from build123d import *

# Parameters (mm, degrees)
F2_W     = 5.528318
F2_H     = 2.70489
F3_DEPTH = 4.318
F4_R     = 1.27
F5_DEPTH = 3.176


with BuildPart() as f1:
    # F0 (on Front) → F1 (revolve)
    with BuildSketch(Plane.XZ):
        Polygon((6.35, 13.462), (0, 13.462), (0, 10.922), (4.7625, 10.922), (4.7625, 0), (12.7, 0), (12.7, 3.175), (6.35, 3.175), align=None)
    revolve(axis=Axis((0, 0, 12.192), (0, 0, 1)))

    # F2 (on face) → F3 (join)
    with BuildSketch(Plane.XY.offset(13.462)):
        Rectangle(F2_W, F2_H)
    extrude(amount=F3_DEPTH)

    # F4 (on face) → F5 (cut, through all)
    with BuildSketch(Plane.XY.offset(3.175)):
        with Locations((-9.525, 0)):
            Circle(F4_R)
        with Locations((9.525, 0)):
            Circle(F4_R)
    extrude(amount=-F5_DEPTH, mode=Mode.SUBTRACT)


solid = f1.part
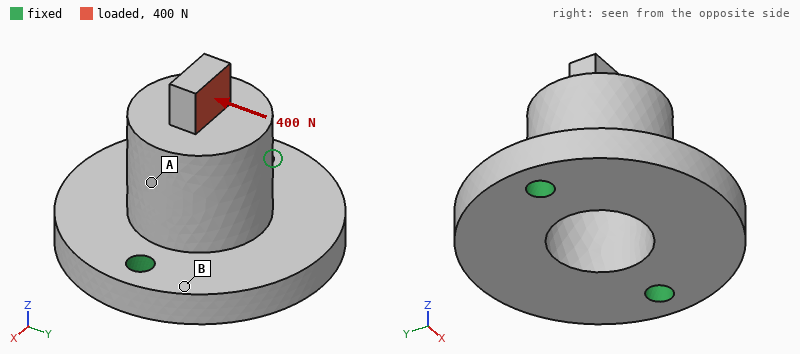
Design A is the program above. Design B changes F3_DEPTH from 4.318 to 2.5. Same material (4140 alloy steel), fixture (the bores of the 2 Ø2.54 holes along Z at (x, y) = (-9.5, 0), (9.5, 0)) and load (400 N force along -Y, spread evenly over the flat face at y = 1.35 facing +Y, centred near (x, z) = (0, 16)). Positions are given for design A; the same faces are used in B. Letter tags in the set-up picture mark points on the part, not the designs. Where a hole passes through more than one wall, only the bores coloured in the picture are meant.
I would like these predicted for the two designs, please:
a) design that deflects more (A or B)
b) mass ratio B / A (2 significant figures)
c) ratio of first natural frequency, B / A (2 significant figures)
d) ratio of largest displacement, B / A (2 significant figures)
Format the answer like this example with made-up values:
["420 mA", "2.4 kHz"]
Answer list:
["A", "0.99", "1.0", "0.76"]
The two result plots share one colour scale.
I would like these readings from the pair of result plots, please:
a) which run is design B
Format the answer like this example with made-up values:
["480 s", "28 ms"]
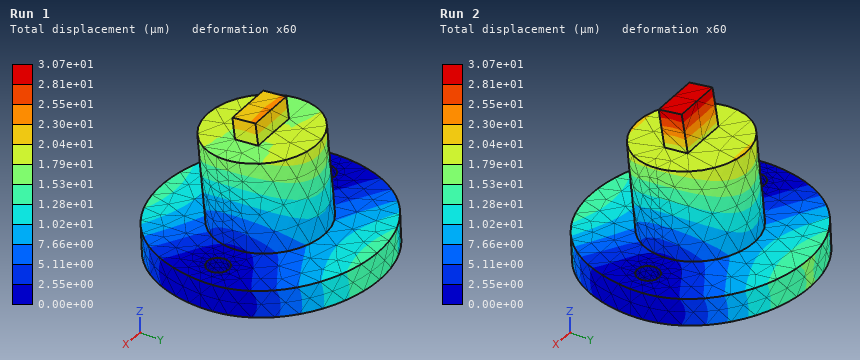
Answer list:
["Run 1"]
